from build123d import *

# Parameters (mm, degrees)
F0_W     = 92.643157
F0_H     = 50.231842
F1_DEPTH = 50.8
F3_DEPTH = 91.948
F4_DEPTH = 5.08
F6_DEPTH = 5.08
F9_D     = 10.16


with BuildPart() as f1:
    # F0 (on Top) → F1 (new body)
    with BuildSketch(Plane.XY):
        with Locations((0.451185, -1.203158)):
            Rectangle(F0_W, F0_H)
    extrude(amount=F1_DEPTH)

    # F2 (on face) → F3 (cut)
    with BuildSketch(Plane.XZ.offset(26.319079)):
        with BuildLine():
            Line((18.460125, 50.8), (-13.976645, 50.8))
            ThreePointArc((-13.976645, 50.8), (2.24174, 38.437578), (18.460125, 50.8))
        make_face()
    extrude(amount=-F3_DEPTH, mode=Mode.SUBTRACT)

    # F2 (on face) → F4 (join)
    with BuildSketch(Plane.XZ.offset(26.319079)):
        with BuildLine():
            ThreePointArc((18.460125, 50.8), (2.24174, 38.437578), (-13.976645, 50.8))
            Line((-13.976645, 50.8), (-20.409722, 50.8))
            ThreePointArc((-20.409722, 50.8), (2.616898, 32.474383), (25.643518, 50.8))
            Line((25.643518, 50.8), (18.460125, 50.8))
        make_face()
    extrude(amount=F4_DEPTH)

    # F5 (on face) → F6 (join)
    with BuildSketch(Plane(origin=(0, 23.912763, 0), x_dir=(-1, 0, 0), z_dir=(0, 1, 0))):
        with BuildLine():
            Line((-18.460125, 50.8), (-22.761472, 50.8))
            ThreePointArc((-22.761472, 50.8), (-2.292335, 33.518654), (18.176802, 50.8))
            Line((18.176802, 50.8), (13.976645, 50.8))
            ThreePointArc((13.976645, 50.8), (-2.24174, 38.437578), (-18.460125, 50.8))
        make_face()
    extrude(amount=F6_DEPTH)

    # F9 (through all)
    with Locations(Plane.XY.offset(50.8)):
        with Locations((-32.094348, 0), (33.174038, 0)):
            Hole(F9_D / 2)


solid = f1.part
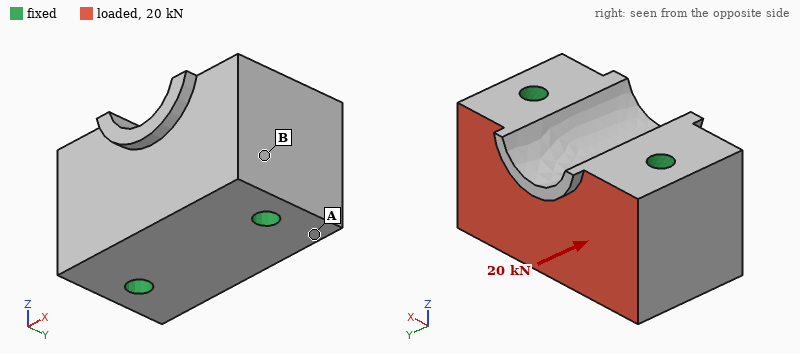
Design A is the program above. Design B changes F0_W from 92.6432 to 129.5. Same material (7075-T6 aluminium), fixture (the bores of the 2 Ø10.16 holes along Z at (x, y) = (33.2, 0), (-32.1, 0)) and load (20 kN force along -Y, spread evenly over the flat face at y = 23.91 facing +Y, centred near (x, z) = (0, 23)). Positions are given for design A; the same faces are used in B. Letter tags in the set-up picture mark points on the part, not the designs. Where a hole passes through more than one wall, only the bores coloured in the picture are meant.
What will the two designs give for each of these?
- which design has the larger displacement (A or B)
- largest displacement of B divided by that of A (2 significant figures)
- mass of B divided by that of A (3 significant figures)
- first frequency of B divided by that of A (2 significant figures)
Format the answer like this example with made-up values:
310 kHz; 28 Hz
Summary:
B; 1.1; 1.44; 0.71
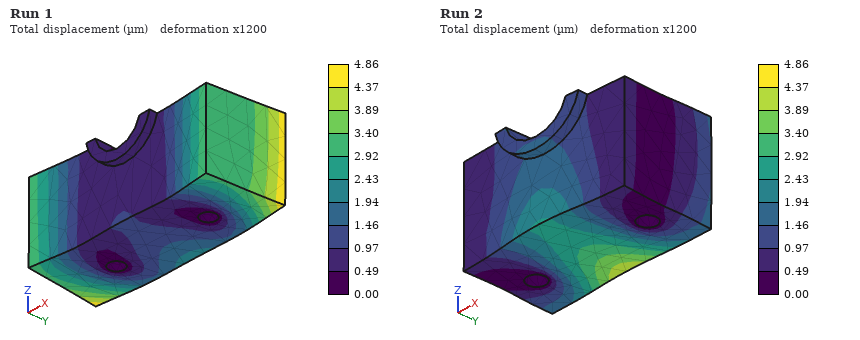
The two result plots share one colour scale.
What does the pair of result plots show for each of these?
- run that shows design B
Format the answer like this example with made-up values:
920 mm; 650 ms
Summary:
Run 1
